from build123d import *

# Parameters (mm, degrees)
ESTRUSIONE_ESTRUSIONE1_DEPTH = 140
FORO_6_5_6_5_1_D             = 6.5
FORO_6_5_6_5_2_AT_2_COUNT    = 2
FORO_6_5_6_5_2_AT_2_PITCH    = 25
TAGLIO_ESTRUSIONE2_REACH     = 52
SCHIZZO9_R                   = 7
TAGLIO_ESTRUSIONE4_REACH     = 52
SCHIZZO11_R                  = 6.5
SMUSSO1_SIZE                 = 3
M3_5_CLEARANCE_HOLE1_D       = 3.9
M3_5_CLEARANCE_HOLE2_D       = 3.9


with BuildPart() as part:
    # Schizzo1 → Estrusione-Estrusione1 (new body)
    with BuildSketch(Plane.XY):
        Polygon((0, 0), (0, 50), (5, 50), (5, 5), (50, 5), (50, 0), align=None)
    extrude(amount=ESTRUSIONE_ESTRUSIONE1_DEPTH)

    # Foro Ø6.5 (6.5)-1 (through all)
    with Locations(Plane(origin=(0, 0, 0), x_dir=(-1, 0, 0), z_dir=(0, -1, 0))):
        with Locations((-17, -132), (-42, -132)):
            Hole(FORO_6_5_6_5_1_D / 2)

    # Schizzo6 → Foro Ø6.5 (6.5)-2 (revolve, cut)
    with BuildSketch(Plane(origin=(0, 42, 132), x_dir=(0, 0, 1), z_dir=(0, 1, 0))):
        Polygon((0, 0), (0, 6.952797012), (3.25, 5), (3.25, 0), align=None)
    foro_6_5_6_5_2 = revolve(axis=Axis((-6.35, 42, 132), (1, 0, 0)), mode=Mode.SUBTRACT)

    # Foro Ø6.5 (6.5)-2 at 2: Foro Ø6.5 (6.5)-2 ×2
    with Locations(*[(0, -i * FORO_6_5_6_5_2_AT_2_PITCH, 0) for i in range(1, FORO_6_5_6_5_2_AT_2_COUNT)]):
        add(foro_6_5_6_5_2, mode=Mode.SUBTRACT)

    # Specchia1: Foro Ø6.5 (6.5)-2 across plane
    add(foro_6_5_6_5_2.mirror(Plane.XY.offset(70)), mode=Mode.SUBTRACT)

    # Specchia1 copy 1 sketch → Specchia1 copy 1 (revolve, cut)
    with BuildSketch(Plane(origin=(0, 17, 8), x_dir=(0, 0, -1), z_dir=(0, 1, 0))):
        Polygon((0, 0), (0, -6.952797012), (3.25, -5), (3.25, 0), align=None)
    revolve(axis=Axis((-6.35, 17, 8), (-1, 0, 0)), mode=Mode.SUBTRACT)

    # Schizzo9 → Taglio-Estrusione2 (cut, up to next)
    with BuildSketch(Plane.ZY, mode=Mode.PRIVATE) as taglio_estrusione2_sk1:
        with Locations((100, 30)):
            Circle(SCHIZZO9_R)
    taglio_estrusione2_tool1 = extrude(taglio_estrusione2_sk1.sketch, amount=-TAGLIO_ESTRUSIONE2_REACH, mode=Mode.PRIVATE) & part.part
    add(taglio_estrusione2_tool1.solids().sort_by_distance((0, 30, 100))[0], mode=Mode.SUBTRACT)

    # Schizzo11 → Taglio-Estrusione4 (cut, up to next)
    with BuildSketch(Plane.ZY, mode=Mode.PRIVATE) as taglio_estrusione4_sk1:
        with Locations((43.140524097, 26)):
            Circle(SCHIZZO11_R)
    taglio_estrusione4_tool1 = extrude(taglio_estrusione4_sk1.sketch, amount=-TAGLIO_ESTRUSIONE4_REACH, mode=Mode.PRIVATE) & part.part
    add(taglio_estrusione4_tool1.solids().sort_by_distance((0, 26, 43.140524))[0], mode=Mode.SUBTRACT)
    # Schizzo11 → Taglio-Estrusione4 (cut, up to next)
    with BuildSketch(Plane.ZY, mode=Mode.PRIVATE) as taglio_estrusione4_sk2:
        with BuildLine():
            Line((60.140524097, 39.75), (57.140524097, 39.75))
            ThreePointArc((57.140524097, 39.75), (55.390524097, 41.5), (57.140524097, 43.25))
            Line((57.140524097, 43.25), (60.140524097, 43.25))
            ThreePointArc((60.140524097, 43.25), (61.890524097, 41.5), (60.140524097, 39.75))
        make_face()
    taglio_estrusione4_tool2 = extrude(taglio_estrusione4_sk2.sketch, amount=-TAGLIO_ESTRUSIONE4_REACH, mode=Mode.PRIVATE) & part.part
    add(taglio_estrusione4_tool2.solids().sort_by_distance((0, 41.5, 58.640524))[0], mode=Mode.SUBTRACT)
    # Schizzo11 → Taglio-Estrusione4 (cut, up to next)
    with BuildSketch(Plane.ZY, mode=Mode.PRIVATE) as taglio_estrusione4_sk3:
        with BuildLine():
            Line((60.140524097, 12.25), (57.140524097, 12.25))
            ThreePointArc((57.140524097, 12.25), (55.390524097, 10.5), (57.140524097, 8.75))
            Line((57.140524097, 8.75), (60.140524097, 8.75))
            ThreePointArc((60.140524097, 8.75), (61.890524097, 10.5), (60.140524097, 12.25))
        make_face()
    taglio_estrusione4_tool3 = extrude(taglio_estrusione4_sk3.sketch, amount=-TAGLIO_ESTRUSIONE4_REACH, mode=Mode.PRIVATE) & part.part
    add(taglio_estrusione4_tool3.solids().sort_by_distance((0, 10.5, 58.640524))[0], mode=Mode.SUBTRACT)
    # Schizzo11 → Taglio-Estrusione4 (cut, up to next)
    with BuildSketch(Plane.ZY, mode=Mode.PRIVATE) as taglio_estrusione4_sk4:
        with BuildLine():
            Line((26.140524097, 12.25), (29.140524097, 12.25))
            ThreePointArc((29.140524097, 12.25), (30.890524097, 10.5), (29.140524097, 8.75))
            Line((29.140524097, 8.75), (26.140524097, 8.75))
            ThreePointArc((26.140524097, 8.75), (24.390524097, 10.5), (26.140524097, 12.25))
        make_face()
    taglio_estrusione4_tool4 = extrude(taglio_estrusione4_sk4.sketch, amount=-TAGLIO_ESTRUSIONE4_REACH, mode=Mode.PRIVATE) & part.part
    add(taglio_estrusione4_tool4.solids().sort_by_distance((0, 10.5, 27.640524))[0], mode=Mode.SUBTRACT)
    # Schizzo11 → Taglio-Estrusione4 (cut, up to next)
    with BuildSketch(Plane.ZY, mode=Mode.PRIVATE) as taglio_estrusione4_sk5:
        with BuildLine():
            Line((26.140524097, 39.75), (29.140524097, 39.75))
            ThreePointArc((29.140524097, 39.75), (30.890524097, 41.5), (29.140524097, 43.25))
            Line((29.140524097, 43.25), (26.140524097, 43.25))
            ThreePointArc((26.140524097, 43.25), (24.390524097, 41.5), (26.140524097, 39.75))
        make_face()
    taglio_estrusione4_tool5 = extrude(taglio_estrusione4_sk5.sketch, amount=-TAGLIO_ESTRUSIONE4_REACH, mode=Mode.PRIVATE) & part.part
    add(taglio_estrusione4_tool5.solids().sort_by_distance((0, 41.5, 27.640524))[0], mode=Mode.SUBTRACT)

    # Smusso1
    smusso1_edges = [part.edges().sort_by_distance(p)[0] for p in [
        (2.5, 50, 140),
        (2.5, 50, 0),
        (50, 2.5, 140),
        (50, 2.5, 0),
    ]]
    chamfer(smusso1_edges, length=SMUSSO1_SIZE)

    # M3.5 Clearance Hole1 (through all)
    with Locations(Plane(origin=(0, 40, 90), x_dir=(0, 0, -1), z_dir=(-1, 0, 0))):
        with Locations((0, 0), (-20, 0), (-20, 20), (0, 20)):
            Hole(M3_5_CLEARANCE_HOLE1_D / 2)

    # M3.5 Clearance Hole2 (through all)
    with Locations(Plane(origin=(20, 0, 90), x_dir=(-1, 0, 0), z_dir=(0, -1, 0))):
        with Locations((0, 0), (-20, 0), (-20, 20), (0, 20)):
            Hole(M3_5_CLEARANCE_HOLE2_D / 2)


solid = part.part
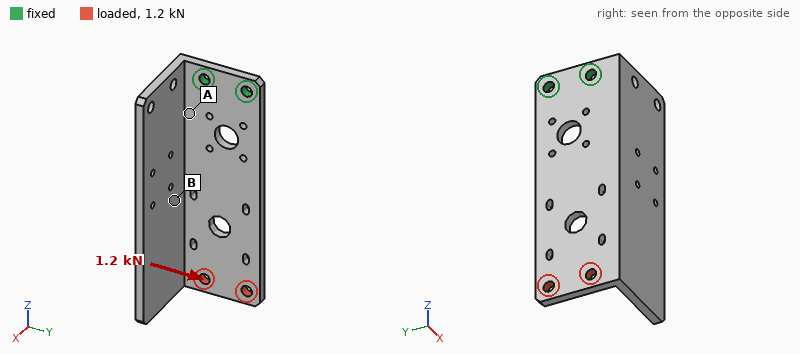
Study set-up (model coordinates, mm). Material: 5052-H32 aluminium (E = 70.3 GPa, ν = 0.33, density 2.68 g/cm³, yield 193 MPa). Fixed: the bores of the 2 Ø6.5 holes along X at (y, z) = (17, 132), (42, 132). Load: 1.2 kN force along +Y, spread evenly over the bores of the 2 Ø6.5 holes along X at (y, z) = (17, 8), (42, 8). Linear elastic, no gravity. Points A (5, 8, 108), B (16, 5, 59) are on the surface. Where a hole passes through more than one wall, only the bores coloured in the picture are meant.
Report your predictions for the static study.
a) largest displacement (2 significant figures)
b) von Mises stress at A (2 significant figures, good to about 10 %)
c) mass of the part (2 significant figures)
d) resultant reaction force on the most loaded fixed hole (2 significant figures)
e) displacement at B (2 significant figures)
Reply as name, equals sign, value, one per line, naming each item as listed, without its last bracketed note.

largest displacement = 0.31 mm
von Mises stress at A = 24 MPa
mass of the part = 170 g
resultant reaction force on the most loaded fixed hole = 5.1 kN
displacement at B = 0.14 mm
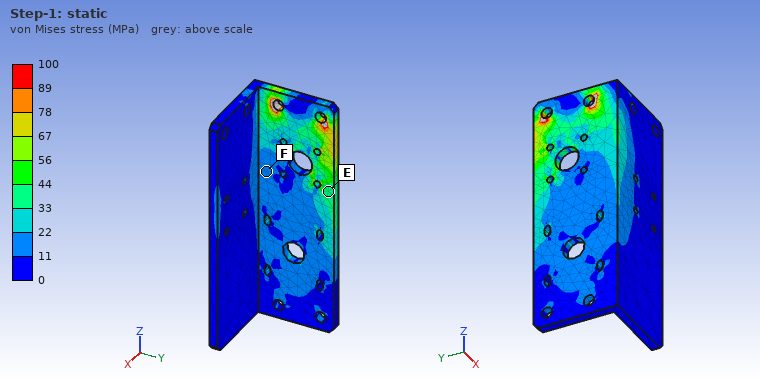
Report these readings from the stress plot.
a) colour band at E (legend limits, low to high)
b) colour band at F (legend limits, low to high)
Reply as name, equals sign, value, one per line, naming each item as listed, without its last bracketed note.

colour band at E = 33 to 44 MPa
colour band at F = 11 to 22 MPa
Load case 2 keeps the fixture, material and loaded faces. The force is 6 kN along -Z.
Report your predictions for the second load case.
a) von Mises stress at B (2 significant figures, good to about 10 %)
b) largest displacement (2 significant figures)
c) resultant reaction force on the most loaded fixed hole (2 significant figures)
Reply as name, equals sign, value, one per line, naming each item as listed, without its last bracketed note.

von Mises stress at B = 6.8 MPa
largest displacement = 0.12 mm
resultant reaction force on the most loaded fixed hole = 3.1 kN
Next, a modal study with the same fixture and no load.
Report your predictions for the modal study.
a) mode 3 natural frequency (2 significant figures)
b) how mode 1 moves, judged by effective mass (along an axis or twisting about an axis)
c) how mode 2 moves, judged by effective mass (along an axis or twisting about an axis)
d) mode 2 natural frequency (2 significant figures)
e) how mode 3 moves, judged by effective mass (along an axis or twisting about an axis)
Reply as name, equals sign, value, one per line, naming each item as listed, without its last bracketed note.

mode 3 natural frequency = 1500 Hz
how mode 1 moves, judged by effective mass = along X
how mode 2 moves, judged by effective mass = along Y
mode 2 natural frequency = 620 Hz
how mode 3 moves, judged by effective mass = along Y
